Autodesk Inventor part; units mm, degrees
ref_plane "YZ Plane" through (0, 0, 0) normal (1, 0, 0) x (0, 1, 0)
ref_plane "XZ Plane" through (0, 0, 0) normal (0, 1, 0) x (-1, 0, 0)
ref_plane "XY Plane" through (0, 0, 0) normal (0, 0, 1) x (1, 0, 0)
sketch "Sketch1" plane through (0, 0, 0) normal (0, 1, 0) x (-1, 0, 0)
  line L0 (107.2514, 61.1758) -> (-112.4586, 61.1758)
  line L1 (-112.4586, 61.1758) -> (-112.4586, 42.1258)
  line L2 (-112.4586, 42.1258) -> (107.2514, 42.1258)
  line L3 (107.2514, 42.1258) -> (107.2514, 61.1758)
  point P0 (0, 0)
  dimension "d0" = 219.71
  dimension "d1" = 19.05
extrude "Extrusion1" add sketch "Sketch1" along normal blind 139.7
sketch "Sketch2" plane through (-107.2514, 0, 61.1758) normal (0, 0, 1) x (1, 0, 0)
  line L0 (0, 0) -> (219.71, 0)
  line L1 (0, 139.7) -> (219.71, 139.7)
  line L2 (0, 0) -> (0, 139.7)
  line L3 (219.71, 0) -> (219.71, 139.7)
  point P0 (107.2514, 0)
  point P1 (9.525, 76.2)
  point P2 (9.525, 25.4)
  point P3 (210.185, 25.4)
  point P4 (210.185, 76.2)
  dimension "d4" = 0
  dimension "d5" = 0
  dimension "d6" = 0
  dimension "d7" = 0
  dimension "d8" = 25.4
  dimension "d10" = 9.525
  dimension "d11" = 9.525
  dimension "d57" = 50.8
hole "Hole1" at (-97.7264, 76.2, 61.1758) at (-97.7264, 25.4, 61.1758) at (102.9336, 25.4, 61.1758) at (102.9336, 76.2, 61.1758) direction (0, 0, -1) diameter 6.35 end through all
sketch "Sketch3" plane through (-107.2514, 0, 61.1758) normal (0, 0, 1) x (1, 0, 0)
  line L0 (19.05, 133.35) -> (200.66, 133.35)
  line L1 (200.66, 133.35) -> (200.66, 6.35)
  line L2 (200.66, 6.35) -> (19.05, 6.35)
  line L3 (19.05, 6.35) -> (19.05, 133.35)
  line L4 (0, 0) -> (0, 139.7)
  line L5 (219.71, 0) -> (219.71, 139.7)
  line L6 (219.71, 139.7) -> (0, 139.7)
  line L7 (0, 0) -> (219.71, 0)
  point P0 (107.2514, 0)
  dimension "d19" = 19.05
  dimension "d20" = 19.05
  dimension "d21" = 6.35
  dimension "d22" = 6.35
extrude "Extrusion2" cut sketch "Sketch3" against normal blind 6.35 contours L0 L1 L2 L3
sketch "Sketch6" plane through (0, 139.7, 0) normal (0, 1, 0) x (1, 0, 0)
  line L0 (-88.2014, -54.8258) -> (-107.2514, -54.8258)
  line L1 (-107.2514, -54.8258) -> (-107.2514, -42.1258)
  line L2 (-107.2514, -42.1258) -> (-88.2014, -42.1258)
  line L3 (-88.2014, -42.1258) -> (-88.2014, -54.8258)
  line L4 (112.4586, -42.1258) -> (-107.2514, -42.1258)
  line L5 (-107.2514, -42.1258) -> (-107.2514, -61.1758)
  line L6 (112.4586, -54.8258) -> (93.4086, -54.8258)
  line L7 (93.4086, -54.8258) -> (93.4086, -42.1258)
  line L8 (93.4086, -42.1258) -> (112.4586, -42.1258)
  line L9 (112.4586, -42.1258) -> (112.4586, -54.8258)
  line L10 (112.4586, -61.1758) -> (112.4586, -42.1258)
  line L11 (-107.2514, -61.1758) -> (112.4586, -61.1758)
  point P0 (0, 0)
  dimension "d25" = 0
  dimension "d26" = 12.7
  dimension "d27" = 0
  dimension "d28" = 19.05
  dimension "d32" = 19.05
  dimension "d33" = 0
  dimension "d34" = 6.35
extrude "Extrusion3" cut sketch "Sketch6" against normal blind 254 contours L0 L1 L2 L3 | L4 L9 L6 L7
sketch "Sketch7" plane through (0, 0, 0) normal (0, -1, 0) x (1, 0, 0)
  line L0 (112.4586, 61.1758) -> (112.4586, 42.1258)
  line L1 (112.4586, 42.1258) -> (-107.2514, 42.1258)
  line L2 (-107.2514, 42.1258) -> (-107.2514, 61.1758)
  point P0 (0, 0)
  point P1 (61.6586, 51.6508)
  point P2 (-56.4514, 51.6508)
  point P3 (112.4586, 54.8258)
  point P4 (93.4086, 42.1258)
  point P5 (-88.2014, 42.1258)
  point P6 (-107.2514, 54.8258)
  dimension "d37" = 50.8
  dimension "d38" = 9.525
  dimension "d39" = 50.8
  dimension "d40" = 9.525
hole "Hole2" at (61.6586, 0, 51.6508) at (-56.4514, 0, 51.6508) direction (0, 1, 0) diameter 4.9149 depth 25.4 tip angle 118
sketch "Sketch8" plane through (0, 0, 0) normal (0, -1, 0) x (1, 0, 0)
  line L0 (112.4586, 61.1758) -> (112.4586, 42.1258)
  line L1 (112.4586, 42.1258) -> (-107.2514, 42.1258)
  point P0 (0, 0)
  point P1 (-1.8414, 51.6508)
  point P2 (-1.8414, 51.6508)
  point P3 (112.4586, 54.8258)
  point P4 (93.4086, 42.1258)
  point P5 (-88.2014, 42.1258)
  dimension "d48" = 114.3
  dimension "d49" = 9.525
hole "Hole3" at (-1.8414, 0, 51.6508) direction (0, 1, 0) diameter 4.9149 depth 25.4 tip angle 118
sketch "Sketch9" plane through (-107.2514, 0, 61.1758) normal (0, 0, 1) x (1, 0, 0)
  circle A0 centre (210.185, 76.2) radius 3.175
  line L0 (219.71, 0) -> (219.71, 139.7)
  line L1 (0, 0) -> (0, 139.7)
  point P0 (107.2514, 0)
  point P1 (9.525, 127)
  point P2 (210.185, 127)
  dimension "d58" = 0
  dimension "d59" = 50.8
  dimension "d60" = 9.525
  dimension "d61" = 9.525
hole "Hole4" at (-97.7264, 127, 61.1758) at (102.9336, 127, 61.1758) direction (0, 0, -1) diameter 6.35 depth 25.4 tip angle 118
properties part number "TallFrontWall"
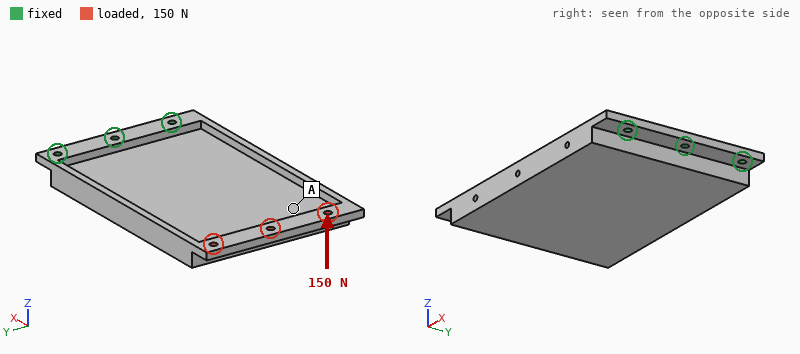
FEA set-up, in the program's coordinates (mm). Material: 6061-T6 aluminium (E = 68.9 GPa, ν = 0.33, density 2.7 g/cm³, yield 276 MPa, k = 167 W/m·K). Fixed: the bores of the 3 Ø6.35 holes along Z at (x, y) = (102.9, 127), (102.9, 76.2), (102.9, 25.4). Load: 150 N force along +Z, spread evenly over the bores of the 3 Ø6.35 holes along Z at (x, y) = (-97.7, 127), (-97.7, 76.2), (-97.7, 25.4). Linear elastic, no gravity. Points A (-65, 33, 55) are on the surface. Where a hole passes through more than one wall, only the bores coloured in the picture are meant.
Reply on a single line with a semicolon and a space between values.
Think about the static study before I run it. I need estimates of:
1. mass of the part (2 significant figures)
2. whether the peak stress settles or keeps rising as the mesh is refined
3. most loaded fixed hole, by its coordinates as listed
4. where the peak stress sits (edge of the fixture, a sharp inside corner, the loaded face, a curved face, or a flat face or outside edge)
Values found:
990 g; keeps rising; (102.9, 76.2); a sharp inside corner
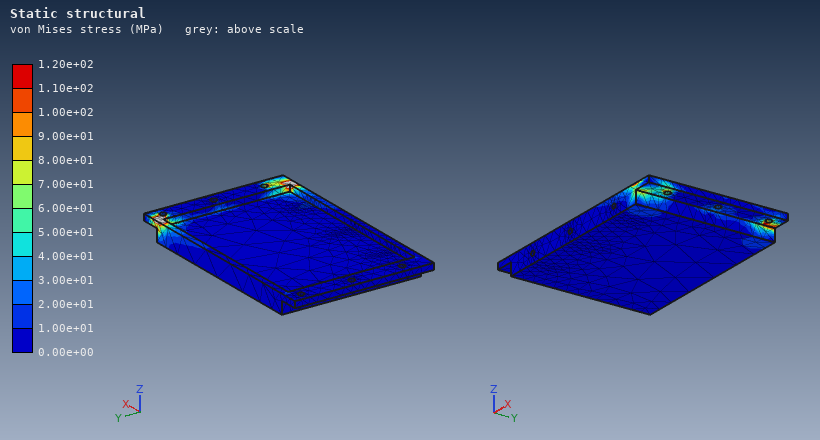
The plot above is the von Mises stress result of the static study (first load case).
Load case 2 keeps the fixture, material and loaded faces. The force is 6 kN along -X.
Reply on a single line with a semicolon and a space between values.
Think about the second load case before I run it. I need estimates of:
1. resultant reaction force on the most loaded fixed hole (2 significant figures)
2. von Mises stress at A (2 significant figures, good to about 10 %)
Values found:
2.3 kN; 14 MPa
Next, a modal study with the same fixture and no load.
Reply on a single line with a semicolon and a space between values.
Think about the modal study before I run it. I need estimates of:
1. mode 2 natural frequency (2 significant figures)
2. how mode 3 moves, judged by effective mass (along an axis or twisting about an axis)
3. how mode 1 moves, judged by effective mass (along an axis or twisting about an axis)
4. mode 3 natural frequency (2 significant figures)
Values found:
630 Hz; along Y; along Z; 1200 Hz
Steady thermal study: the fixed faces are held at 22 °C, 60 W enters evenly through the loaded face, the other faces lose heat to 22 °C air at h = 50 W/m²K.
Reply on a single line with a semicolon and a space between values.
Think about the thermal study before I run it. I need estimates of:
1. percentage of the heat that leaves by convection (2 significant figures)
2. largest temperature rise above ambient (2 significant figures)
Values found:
74 %; 35 K
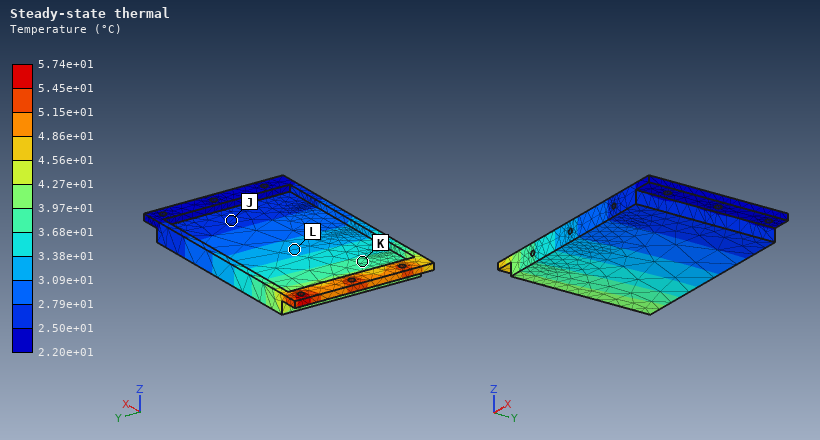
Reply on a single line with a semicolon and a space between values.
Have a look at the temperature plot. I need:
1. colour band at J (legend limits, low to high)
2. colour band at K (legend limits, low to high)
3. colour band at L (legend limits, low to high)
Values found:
2.50e+01 to 2.79e+01 °C; 3.68e+01 to 3.97e+01 °C; 3.09e+01 to 3.38e+01 °C
